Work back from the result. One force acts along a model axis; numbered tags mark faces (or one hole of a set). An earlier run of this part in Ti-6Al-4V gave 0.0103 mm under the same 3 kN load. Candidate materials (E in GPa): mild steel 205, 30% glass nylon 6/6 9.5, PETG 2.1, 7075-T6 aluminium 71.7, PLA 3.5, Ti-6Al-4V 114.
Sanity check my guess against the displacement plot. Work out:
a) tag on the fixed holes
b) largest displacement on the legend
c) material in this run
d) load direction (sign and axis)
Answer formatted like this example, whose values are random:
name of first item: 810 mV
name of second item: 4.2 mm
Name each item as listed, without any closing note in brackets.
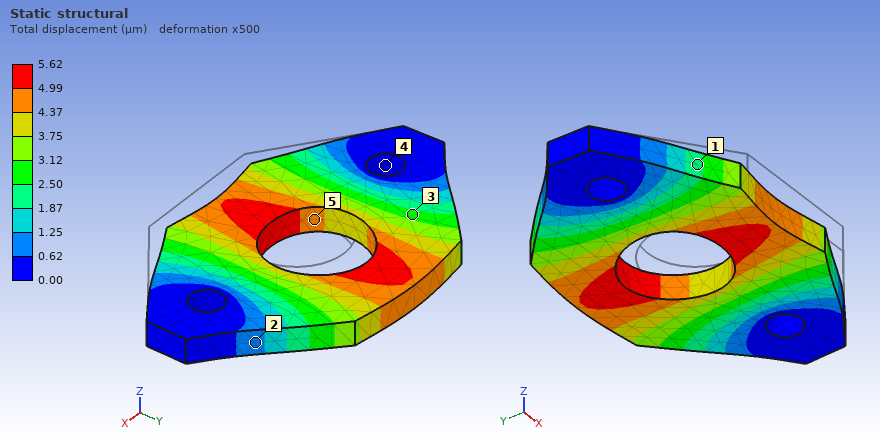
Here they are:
tag on the fixed holes: 4
largest displacement on the legend: 5.62 µm
material in this run: mild steel
load direction: +Y
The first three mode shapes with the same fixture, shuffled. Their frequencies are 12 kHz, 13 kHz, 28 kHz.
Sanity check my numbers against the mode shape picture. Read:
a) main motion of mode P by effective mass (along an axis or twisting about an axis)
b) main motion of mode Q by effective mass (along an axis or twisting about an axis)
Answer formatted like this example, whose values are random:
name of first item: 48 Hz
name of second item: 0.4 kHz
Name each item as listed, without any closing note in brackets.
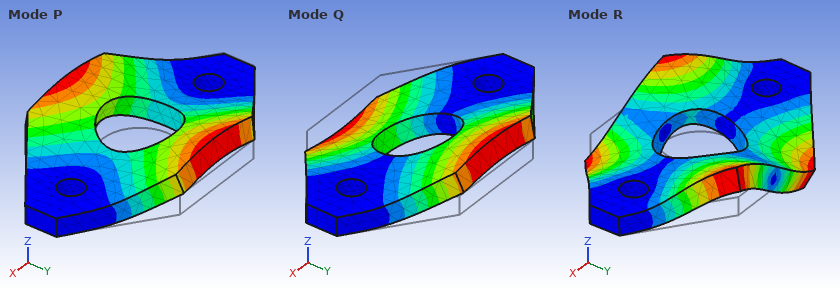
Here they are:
main motion of mode P by effective mass: along Z
main motion of mode Q by effective mass: twisting about X
